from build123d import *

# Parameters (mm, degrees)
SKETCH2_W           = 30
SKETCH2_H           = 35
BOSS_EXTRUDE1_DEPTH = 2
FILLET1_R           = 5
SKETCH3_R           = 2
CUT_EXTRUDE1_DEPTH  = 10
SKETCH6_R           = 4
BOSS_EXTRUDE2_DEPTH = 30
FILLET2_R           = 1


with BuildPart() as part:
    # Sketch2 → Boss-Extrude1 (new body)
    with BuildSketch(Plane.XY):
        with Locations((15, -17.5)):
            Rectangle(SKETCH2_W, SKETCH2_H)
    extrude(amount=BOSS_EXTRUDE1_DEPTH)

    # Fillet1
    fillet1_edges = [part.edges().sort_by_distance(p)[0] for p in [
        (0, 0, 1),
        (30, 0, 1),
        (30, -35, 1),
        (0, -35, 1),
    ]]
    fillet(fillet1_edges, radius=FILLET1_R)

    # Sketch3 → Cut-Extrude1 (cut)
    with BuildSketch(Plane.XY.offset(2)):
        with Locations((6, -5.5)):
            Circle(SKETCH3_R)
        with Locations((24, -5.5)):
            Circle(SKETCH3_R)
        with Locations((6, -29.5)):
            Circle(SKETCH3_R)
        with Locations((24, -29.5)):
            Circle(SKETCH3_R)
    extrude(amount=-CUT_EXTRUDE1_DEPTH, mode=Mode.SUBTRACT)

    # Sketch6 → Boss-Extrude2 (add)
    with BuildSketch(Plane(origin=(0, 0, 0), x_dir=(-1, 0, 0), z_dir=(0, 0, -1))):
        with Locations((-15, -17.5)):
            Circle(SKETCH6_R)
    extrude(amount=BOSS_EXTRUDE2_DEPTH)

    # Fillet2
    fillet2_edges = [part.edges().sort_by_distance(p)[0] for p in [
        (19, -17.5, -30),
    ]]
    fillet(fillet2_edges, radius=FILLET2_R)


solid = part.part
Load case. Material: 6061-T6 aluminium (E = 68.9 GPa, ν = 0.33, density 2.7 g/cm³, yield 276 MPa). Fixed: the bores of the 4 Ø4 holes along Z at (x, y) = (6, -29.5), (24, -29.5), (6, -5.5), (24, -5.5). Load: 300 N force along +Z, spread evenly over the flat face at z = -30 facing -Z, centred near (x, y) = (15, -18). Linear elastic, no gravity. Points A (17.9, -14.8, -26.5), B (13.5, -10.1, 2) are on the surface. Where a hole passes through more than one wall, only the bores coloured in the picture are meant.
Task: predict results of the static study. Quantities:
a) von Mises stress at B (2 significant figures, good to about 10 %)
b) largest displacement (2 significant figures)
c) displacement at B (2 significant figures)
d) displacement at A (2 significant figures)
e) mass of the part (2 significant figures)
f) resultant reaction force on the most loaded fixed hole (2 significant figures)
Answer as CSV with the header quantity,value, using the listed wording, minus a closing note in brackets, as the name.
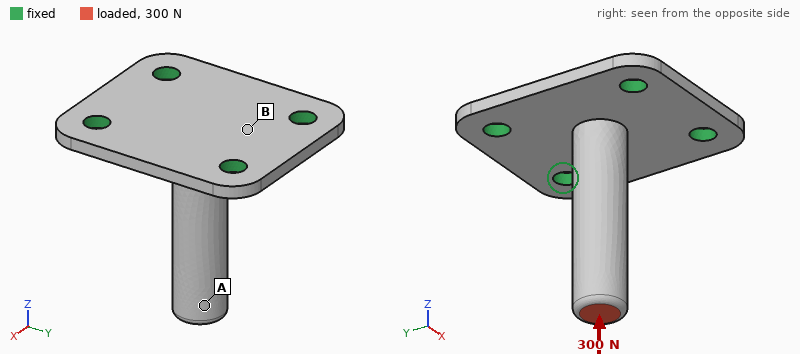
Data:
quantity,value
von Mises stress at B,19 MPa
largest displacement,19 µm
displacement at B,9.7 µm
displacement at A,18 µm
mass of the part,9.3 g
resultant reaction force on the most loaded fixed hole,77 N
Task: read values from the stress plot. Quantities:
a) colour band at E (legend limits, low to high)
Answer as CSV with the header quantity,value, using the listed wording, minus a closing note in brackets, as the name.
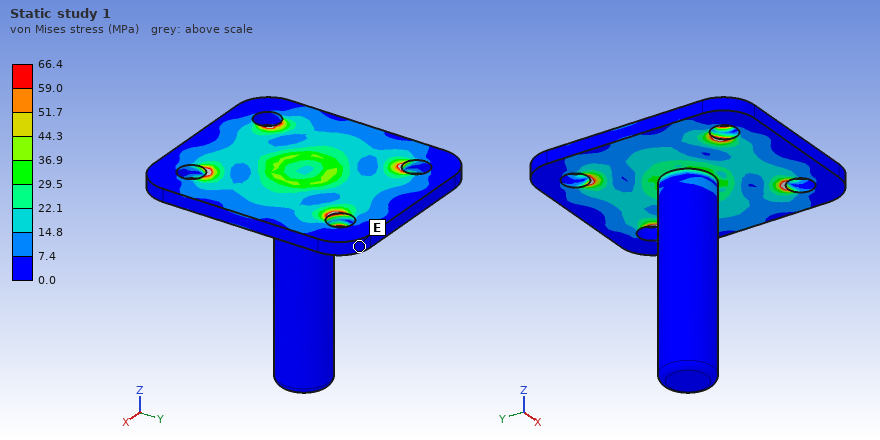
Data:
quantity,value
colour band at E,0.0 to 7.4 MPa
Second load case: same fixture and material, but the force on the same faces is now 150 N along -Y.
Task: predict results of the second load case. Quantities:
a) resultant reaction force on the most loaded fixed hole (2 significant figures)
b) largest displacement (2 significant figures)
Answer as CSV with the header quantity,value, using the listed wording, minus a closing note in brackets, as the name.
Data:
quantity,value
resultant reaction force on the most loaded fixed hole,140 N
largest displacement,0.26 mm
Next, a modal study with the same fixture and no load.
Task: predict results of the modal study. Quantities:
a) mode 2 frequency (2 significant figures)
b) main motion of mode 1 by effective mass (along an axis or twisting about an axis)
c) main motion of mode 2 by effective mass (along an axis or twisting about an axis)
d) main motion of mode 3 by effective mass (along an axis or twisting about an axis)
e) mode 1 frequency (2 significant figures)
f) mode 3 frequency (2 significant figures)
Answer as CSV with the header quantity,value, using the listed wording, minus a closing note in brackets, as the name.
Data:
quantity,value
mode 2 frequency,3400 Hz
main motion of mode 1 by effective mass,along X
main motion of mode 2 by effective mass,along Y
main motion of mode 3 by effective mass,along Z
mode 1 frequency,3200 Hz
mode 3 frequency,9500 Hz
